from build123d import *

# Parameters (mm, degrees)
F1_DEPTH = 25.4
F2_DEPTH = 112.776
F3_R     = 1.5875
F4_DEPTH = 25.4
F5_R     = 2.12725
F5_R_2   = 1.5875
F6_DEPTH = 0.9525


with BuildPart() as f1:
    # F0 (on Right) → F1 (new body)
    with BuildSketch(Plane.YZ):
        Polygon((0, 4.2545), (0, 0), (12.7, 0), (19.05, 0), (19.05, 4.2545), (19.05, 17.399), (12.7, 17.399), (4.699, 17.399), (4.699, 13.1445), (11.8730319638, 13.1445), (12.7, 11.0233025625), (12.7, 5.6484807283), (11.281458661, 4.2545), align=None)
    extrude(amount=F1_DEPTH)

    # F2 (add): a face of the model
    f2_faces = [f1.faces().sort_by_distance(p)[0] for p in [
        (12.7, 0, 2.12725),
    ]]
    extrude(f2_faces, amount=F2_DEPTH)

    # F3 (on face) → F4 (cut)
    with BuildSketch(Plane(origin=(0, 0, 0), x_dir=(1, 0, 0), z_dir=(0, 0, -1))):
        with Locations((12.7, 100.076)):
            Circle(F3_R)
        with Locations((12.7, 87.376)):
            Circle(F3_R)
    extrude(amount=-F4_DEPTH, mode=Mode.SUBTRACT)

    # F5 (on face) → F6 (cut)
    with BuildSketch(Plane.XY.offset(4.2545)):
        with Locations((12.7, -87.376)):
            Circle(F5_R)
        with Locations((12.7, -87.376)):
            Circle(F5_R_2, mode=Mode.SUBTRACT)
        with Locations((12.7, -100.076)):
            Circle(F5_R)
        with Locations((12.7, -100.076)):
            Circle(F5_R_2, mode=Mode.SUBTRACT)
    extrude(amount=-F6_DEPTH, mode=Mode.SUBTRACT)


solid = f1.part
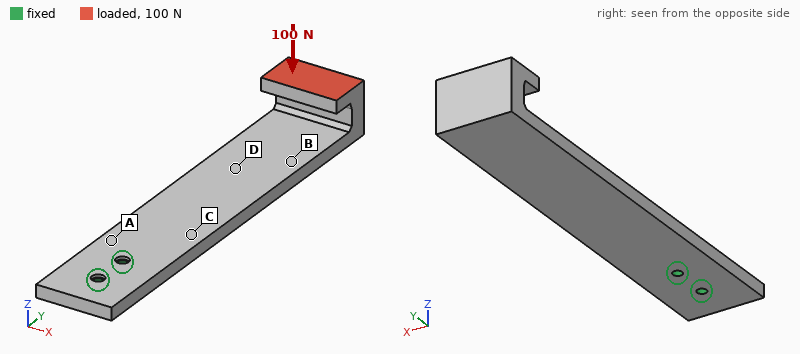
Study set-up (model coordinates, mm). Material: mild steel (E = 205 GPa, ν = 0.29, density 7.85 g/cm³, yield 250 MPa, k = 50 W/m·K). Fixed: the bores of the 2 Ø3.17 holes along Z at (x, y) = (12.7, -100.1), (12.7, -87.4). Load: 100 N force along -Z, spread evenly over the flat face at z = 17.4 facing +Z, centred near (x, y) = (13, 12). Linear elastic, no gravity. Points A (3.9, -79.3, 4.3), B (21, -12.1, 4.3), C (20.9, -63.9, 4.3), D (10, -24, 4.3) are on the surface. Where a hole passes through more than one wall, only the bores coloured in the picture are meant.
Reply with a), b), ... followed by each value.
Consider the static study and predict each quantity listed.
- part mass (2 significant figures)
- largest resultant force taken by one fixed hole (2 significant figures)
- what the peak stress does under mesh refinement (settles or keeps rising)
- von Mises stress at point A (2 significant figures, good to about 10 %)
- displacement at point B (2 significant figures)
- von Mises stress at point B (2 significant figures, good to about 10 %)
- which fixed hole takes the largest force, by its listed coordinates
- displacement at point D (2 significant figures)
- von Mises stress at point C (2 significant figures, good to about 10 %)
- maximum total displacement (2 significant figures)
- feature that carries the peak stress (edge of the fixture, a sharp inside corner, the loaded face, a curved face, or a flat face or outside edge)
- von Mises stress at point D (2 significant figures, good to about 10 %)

a) 140 g
b) 580 N
c) keeps rising
d) 120 MPa
e) 0.67 mm
f) 31 MPa
g) (12.7, -87.4)
h) 0.50 mm
i) 98 MPa
j) 1.2 mm
k) edge of the fixture
l) 47 MPa
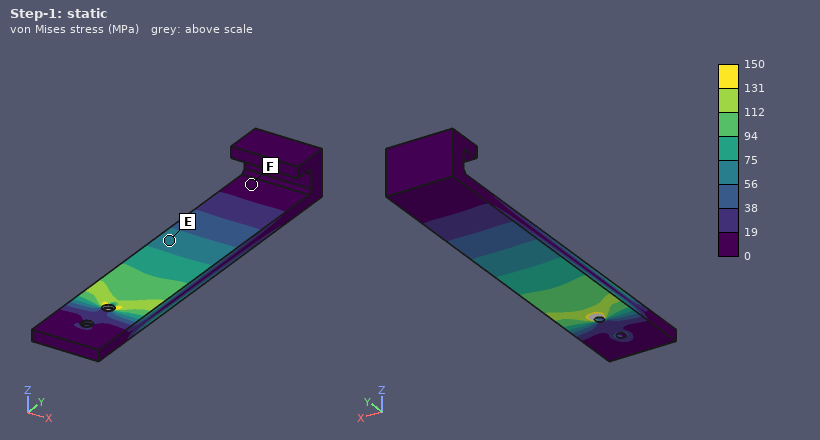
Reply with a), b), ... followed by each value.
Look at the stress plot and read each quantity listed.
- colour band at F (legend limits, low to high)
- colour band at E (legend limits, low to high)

a) 0 to 19 MPa
b) 56 to 75 MPa
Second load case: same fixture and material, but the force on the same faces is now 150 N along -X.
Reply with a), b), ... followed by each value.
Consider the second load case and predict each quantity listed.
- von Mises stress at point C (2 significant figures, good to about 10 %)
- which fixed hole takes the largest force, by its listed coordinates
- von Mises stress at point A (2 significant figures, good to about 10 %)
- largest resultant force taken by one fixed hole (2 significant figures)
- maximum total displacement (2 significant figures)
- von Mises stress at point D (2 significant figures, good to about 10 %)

a) 34 MPa
b) (12.7, -87.4)
c) 30 MPa
d) 1.1 kN
e) 0.16 mm
f) 32 MPa
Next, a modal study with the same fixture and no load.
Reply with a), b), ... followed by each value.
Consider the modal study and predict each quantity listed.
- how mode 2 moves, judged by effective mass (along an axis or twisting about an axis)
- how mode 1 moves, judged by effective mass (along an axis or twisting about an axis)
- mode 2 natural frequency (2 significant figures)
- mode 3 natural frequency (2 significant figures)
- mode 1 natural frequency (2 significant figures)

a) along X
b) along Z
c) 950 Hz
d) 1500 Hz
e) 220 Hz
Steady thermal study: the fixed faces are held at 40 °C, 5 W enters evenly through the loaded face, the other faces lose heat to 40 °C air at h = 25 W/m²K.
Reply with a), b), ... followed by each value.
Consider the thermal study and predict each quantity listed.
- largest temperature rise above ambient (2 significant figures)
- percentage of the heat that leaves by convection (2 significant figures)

a) 46 K
b) 76 %
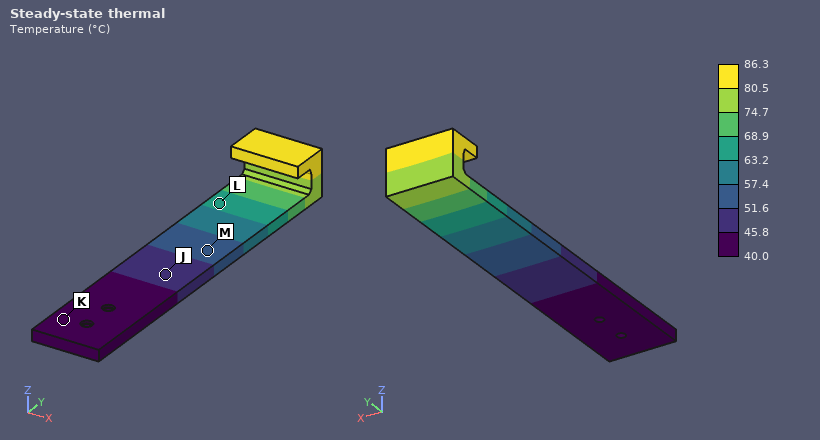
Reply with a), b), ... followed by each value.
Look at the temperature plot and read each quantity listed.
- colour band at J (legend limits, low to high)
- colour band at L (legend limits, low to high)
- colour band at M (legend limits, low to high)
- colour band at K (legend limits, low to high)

a) 45.8 to 51.6 °C
b) 63.2 to 68.9 °C
c) 51.6 to 57.4 °C
d) 40.0 to 45.8 °C
